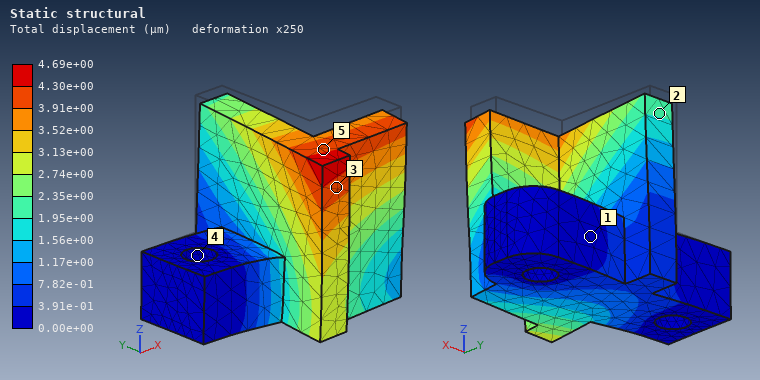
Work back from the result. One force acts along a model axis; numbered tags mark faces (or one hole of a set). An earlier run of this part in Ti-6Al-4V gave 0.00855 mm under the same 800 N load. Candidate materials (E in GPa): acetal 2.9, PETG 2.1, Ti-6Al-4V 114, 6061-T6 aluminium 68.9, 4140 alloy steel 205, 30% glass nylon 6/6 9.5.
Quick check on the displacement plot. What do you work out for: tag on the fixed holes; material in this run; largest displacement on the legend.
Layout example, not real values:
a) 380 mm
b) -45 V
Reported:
a) 4
b) 4140 alloy steel
c) 4.69e+00 µm
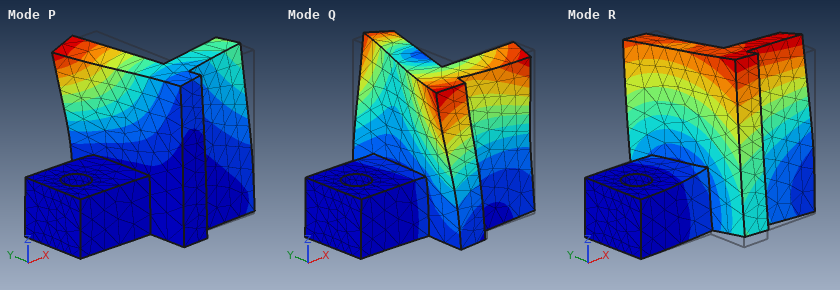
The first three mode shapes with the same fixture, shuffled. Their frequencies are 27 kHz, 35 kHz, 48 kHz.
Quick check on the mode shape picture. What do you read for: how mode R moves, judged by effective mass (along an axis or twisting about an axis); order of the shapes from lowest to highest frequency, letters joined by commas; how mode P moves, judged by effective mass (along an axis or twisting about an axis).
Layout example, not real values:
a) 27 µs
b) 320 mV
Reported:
a) along Y
b) R, P, Q
c) along X
